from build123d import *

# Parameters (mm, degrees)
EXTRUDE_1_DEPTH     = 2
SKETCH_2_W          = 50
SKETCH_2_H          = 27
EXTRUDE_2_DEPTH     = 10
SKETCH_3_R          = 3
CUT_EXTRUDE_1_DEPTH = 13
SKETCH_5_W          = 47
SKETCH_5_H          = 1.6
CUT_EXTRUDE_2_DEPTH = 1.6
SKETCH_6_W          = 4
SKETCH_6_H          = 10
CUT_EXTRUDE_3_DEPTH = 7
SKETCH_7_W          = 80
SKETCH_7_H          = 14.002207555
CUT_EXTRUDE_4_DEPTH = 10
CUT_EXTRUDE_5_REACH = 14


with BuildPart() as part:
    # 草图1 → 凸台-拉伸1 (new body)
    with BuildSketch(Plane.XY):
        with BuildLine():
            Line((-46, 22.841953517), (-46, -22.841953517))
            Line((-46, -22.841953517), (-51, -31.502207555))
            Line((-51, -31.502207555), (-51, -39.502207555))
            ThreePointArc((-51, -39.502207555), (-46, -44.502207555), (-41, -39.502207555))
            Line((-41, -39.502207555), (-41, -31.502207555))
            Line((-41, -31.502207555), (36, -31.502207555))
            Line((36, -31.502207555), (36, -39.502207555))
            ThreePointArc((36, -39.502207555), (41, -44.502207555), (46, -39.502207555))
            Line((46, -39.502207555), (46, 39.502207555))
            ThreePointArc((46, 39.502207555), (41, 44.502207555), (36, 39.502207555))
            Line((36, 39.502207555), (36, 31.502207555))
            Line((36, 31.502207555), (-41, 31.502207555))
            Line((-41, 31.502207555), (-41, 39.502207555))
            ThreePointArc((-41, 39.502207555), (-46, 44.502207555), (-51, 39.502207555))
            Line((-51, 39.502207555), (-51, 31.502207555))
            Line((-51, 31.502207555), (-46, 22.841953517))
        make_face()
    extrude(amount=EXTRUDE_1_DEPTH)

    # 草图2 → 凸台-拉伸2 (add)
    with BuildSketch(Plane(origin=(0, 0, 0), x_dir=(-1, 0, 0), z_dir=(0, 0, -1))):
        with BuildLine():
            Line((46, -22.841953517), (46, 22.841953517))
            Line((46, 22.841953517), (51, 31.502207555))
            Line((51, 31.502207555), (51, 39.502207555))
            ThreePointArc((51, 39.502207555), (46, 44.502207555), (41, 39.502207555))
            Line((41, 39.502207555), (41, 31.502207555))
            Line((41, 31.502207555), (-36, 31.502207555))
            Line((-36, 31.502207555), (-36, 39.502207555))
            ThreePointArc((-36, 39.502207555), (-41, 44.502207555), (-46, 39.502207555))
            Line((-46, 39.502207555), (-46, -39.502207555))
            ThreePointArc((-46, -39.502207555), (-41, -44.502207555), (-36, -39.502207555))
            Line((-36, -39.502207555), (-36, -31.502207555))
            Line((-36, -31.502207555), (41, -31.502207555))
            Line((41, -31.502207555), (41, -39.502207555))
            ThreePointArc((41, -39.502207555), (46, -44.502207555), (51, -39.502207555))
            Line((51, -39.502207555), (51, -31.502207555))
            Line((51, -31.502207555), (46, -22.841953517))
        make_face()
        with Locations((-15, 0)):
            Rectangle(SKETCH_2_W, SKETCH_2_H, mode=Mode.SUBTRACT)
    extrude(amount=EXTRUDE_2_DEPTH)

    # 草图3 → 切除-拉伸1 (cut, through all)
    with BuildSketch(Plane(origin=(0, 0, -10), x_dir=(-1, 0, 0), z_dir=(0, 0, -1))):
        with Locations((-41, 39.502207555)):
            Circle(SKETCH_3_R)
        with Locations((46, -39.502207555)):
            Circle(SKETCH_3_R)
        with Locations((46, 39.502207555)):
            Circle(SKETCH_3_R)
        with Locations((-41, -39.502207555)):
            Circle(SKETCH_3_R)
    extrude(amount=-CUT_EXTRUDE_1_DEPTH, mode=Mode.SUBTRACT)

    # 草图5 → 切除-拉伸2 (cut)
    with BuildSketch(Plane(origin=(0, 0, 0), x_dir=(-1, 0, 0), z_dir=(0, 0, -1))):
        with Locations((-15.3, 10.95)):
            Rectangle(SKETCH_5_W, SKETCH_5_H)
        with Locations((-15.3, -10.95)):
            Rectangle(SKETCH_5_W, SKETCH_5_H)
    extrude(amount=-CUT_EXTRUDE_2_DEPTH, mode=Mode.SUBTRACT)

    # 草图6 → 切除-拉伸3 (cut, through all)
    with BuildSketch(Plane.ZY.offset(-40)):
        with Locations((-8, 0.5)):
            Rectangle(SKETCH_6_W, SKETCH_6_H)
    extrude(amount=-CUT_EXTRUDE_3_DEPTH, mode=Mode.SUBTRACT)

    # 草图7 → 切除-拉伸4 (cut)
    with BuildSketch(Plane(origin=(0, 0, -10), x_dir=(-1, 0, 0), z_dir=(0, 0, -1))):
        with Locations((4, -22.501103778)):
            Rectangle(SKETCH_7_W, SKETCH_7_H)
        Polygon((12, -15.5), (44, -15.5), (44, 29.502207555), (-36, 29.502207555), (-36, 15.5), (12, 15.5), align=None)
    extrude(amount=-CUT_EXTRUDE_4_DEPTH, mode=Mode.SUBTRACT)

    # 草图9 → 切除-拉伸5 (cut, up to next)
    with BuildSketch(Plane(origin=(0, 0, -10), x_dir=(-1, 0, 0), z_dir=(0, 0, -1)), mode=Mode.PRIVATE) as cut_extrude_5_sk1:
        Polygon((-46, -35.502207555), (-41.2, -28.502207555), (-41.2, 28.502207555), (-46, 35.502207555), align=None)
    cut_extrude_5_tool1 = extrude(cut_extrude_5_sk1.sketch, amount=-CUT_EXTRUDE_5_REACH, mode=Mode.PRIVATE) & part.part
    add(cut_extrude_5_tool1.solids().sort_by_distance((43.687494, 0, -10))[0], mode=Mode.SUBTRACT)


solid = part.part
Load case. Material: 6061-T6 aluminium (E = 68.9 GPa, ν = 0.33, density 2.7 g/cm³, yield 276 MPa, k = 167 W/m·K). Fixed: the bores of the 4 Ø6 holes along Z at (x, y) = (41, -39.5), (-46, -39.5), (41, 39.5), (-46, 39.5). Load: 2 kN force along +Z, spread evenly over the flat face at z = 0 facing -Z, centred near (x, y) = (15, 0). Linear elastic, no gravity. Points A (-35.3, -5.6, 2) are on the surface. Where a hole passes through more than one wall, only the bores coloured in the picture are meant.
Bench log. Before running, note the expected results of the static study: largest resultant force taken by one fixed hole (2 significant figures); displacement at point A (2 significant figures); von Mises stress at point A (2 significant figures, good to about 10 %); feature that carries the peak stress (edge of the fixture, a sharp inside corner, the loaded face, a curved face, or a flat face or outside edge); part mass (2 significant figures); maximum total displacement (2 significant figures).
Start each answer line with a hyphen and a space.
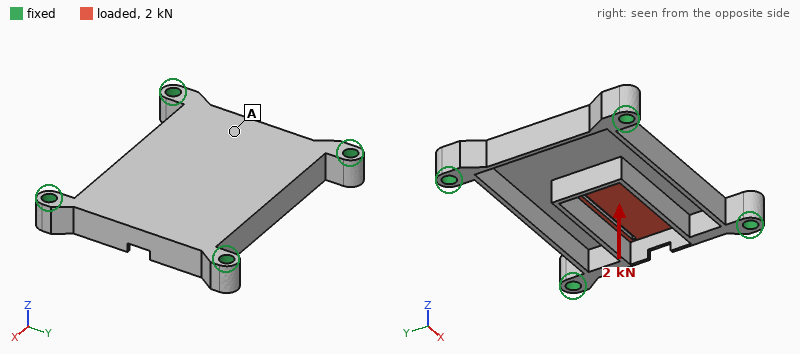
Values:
- 990 N
- 0.093 mm
- 20 MPa
- a flat face or outside edge
- 67 g
- 0.35 mm
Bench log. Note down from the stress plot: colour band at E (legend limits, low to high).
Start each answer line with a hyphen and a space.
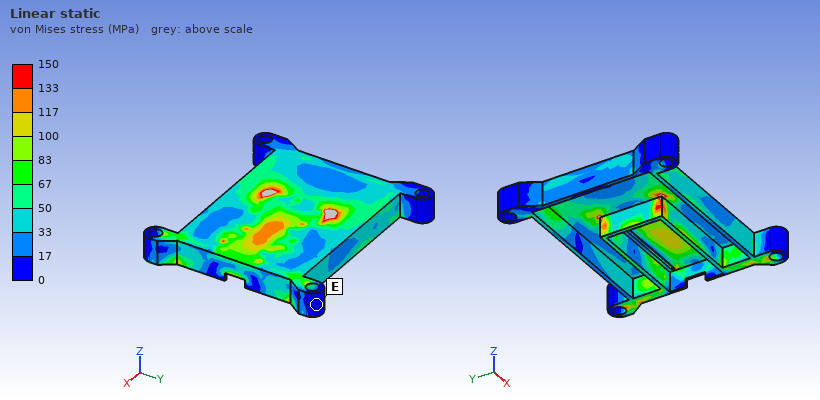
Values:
- 0 to 17 MPa
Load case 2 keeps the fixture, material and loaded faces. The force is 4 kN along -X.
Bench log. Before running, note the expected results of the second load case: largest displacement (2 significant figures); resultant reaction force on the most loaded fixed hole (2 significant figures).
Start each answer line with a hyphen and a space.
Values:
- 38 µm
- 1.1 kN
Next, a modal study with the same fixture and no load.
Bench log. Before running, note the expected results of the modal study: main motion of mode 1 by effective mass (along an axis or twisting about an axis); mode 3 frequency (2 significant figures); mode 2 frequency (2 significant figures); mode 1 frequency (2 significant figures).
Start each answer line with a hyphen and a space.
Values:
- along Z
- 6600 Hz
- 4800 Hz
- 2700 Hz
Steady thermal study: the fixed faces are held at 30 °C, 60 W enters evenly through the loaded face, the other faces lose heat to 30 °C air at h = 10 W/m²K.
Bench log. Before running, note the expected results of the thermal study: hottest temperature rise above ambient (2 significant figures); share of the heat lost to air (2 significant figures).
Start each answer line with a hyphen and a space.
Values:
- 56 K
- 8.1 %
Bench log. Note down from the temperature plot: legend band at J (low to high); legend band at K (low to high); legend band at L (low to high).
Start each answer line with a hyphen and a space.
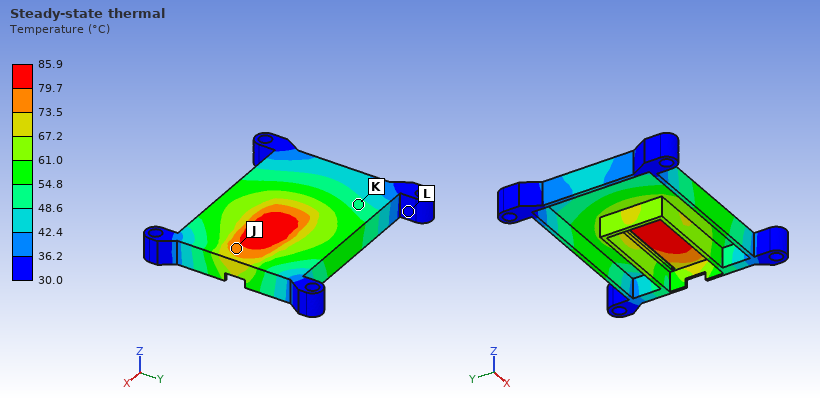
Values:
- 73.5 to 79.7 °C
- 48.6 to 54.8 °C
- 30.0 to 36.2 °C
